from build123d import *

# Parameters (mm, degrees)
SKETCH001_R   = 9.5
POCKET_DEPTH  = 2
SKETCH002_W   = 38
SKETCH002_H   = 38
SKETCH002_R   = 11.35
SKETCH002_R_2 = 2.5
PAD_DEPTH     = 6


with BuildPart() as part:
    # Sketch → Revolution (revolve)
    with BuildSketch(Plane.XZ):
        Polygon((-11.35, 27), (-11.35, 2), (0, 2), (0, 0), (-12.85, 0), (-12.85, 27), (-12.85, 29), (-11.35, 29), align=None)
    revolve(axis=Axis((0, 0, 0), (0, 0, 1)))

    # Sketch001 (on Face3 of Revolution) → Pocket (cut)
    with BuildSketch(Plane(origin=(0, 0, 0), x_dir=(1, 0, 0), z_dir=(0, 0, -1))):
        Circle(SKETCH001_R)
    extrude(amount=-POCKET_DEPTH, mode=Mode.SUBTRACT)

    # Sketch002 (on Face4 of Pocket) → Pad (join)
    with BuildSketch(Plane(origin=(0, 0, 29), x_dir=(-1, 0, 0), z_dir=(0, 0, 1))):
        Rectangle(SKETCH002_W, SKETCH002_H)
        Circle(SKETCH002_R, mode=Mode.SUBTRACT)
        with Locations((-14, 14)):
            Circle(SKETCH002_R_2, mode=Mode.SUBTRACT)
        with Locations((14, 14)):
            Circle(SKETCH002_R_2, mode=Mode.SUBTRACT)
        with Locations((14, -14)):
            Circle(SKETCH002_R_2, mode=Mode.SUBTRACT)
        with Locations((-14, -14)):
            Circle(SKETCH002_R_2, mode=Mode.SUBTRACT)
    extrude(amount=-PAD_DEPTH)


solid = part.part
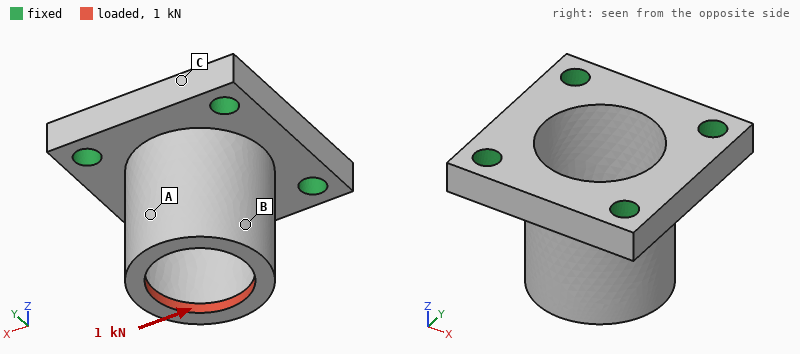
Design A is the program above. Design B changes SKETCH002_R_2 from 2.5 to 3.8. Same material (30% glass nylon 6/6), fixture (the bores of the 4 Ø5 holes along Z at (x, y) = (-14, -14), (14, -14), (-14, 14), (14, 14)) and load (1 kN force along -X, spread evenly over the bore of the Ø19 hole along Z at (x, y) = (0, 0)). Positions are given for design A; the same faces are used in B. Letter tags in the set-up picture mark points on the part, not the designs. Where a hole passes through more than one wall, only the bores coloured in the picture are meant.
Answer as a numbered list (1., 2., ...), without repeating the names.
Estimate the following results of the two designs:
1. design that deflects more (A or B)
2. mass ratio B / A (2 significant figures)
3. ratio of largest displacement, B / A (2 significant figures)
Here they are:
1. A
2. 0.93
3. 0.90
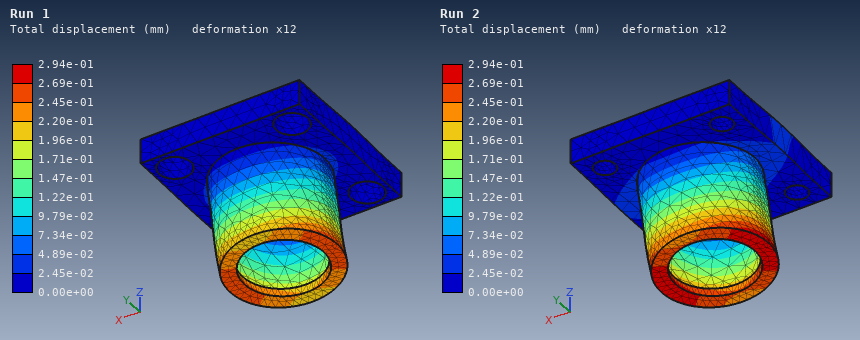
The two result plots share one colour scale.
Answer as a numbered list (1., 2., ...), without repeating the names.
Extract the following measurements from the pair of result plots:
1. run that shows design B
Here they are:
1. Run 1
